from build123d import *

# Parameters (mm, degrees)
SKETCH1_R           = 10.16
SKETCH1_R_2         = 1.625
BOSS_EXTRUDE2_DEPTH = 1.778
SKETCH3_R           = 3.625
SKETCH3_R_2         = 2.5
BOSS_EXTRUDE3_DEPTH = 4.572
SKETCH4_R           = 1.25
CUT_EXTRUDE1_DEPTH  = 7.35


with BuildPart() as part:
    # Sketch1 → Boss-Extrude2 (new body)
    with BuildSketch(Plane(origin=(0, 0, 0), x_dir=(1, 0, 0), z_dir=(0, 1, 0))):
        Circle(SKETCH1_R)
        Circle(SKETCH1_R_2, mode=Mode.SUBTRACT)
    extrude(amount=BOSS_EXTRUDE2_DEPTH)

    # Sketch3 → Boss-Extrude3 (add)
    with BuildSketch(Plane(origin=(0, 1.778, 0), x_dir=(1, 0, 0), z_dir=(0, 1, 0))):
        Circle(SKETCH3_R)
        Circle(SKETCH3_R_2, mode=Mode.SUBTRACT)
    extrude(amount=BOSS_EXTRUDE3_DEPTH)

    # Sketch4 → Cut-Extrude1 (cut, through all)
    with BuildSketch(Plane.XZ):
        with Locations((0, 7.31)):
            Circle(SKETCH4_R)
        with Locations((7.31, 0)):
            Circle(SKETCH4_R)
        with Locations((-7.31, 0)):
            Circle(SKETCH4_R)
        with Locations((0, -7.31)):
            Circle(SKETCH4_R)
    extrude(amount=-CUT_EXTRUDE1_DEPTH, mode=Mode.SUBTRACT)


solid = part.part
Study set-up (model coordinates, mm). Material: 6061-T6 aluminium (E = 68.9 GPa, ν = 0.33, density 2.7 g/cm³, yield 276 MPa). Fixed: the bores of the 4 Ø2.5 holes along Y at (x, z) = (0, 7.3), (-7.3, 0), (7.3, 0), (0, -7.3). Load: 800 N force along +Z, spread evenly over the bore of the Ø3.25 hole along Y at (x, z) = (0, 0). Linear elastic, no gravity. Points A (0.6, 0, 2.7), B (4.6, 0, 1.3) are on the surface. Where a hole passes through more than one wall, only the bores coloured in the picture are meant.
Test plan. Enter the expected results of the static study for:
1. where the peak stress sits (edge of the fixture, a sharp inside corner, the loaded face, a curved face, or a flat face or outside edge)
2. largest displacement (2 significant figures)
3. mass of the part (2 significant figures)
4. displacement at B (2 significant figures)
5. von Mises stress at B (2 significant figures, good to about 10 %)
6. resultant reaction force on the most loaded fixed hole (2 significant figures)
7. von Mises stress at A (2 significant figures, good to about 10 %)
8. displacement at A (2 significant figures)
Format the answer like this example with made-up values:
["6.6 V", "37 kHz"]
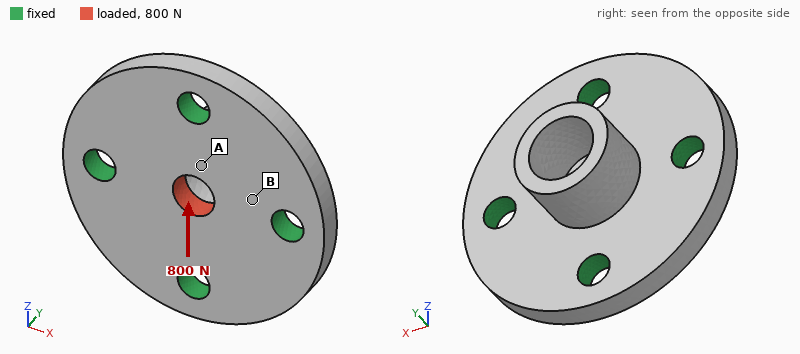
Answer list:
["the loaded face", "2.9 µm", "1.7 g", "0.82 µm", "9.7 MPa", "270 N", "45 MPa", "2.0 µm"]
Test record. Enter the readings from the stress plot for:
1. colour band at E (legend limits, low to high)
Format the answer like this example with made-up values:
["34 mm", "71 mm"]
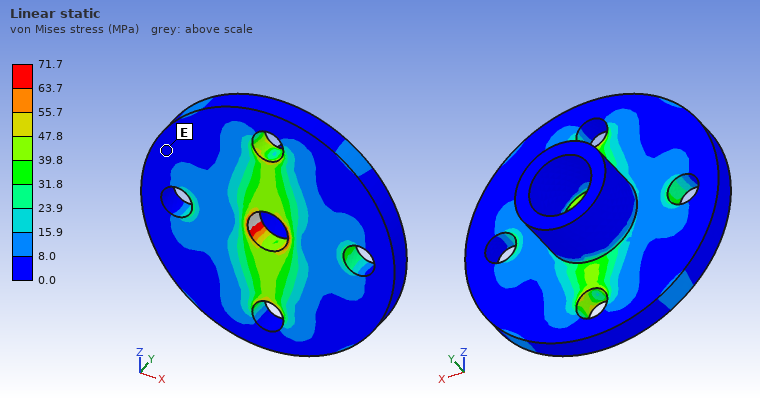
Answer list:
["0.0 to 8.0 MPa"]
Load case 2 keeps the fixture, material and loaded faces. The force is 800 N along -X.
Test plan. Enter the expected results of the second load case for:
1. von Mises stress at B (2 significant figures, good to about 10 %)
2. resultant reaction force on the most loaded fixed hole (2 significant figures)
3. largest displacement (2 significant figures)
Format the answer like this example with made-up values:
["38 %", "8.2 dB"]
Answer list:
["31 MPa", "270 N", "2.9 µm"]
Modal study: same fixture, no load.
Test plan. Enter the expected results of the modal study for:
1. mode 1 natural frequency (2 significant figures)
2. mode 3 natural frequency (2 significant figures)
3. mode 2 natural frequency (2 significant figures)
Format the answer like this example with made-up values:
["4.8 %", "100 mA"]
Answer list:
["62 kHz", "62 kHz", "62 kHz"]
